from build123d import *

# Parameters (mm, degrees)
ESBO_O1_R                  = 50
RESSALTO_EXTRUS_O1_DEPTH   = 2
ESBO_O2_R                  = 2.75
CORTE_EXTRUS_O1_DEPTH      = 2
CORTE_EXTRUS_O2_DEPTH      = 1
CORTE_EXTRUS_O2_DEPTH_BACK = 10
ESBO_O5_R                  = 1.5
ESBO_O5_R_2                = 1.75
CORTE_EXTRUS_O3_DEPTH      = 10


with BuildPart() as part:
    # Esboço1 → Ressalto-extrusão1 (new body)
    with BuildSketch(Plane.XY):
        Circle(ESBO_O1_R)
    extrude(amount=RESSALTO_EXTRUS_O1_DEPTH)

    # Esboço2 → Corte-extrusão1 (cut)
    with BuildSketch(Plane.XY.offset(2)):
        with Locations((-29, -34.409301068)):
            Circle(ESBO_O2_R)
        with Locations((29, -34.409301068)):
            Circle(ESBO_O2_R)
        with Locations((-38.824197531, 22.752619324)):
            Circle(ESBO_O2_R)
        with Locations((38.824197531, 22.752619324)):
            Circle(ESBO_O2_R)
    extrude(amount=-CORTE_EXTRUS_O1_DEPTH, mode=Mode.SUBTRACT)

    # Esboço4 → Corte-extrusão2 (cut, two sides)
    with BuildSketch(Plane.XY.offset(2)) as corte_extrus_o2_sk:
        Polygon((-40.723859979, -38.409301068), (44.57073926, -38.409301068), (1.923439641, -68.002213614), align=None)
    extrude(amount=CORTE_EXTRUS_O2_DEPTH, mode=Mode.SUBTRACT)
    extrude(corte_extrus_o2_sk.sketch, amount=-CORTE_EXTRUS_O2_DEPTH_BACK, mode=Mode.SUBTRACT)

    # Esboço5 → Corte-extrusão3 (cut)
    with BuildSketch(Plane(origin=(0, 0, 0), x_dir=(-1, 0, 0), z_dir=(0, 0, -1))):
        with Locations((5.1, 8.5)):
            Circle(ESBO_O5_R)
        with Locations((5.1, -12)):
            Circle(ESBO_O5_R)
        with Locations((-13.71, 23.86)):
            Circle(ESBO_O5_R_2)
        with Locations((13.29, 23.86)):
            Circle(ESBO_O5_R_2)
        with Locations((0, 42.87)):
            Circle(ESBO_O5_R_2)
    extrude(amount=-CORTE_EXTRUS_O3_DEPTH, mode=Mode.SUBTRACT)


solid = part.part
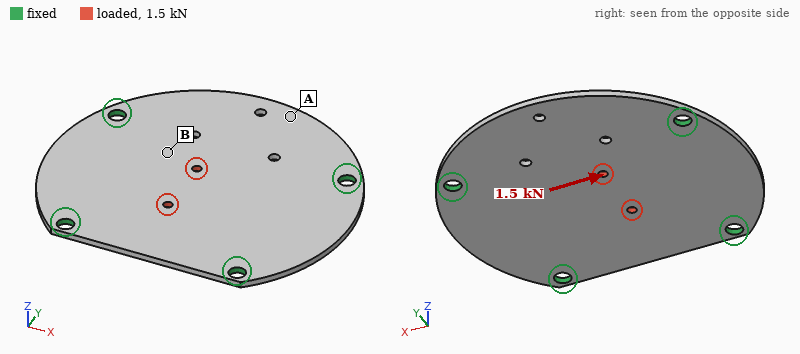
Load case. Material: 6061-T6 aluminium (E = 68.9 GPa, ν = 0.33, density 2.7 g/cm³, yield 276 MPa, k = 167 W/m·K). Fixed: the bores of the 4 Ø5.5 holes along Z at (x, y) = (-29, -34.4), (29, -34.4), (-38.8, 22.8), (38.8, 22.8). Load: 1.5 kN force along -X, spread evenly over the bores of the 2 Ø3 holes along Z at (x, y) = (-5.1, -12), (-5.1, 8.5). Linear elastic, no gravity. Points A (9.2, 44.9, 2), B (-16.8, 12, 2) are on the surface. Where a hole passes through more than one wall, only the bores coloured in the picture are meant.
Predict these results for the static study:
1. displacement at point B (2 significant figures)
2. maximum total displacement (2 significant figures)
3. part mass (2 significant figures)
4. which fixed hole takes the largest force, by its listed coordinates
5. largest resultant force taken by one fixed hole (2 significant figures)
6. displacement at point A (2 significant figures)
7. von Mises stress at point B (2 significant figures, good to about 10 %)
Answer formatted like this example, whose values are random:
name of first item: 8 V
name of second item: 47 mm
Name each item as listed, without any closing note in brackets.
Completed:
displacement at point B: 4.6 µm
maximum total displacement: 8.1 µm
part mass: 39 g
which fixed hole takes the largest force, by its listed coordinates: (-38.8, 22.8)
largest resultant force taken by one fixed hole: 450 N
displacement at point A: 1.9 µm
von Mises stress at point B: 12 MPa
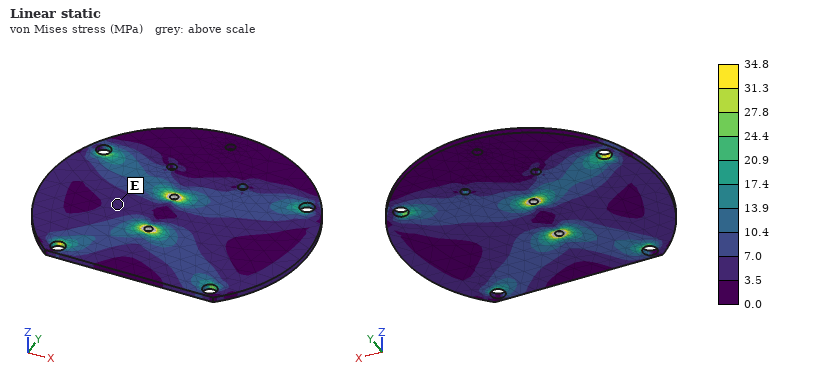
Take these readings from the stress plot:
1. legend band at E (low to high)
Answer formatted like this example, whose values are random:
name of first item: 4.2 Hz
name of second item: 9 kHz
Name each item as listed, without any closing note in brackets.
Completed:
legend band at E: 3.5 to 7.0 MPa
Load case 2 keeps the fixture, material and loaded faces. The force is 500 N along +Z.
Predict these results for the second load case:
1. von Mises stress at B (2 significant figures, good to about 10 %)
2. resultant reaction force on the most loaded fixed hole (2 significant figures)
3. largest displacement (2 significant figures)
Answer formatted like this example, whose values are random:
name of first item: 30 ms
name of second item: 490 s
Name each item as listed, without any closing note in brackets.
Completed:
von Mises stress at B: 40 MPa
resultant reaction force on the most loaded fixed hole: 160 N
largest displacement: 0.44 mm
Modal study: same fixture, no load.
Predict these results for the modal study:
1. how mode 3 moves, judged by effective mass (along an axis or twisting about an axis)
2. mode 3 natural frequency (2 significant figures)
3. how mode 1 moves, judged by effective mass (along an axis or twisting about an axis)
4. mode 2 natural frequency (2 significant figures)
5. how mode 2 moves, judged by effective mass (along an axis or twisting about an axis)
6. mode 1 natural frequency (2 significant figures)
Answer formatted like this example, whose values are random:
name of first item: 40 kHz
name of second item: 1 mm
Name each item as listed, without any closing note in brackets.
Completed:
how mode 3 moves, judged by effective mass: twisting about Y
mode 3 natural frequency: 3100 Hz
how mode 1 moves, judged by effective mass: along Z
mode 2 natural frequency: 2000 Hz
how mode 2 moves, judged by effective mass: along Z
mode 1 natural frequency: 1400 Hz
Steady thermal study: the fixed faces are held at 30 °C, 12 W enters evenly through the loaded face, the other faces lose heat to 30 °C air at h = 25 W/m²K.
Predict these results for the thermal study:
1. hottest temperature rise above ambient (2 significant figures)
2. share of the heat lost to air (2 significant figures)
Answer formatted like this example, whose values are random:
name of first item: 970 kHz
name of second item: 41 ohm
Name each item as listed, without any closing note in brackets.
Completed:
hottest temperature rise above ambient: 15 K
share of the heat lost to air: 15 %
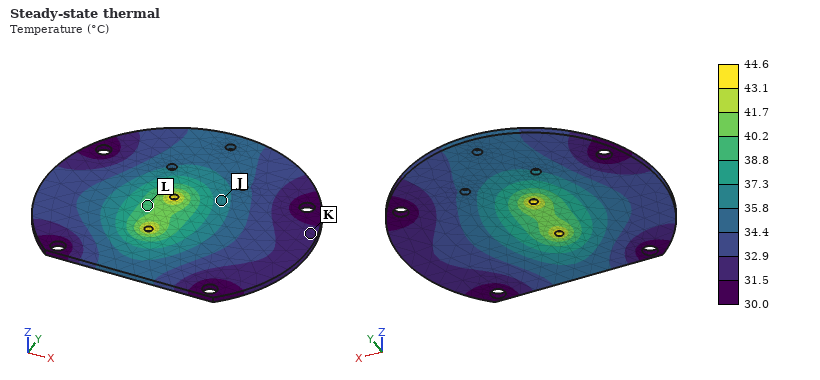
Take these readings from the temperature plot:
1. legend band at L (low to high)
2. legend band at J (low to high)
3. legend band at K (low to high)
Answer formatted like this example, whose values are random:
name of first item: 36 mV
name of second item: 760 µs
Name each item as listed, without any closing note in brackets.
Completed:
legend band at L: 38.8 to 40.2 °C
legend band at J: 35.8 to 37.3 °C
legend band at K: 31.5 to 32.9 °C
